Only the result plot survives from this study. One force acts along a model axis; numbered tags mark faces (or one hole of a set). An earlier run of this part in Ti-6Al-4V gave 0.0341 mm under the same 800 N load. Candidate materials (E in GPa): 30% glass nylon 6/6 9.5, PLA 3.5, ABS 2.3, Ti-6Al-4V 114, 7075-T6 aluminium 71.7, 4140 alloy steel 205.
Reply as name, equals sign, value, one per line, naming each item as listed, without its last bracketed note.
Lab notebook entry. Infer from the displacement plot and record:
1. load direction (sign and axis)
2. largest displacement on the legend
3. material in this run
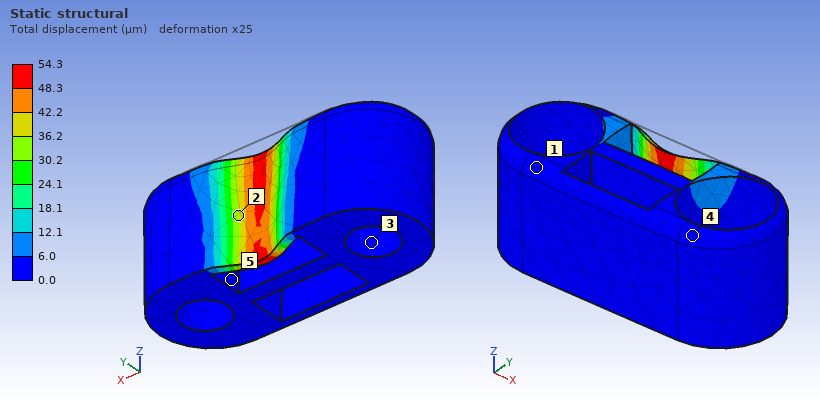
load direction = -Y
largest displacement on the legend = 54.3 µm
material in this run = 7075-T6 aluminium
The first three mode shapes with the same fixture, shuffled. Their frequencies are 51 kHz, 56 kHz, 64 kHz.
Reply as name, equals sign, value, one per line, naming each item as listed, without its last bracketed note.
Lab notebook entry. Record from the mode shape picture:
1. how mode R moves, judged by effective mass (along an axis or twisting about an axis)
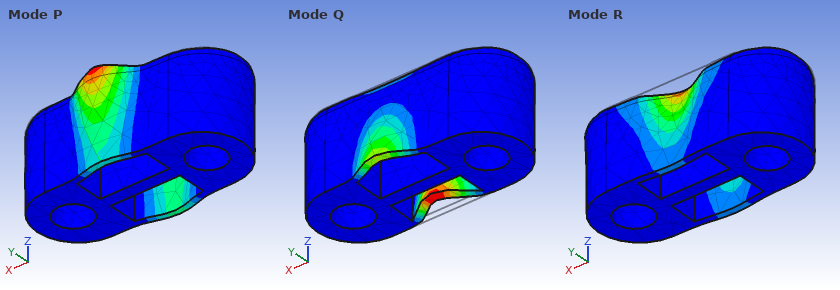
how mode R moves, judged by effective mass = along Y
